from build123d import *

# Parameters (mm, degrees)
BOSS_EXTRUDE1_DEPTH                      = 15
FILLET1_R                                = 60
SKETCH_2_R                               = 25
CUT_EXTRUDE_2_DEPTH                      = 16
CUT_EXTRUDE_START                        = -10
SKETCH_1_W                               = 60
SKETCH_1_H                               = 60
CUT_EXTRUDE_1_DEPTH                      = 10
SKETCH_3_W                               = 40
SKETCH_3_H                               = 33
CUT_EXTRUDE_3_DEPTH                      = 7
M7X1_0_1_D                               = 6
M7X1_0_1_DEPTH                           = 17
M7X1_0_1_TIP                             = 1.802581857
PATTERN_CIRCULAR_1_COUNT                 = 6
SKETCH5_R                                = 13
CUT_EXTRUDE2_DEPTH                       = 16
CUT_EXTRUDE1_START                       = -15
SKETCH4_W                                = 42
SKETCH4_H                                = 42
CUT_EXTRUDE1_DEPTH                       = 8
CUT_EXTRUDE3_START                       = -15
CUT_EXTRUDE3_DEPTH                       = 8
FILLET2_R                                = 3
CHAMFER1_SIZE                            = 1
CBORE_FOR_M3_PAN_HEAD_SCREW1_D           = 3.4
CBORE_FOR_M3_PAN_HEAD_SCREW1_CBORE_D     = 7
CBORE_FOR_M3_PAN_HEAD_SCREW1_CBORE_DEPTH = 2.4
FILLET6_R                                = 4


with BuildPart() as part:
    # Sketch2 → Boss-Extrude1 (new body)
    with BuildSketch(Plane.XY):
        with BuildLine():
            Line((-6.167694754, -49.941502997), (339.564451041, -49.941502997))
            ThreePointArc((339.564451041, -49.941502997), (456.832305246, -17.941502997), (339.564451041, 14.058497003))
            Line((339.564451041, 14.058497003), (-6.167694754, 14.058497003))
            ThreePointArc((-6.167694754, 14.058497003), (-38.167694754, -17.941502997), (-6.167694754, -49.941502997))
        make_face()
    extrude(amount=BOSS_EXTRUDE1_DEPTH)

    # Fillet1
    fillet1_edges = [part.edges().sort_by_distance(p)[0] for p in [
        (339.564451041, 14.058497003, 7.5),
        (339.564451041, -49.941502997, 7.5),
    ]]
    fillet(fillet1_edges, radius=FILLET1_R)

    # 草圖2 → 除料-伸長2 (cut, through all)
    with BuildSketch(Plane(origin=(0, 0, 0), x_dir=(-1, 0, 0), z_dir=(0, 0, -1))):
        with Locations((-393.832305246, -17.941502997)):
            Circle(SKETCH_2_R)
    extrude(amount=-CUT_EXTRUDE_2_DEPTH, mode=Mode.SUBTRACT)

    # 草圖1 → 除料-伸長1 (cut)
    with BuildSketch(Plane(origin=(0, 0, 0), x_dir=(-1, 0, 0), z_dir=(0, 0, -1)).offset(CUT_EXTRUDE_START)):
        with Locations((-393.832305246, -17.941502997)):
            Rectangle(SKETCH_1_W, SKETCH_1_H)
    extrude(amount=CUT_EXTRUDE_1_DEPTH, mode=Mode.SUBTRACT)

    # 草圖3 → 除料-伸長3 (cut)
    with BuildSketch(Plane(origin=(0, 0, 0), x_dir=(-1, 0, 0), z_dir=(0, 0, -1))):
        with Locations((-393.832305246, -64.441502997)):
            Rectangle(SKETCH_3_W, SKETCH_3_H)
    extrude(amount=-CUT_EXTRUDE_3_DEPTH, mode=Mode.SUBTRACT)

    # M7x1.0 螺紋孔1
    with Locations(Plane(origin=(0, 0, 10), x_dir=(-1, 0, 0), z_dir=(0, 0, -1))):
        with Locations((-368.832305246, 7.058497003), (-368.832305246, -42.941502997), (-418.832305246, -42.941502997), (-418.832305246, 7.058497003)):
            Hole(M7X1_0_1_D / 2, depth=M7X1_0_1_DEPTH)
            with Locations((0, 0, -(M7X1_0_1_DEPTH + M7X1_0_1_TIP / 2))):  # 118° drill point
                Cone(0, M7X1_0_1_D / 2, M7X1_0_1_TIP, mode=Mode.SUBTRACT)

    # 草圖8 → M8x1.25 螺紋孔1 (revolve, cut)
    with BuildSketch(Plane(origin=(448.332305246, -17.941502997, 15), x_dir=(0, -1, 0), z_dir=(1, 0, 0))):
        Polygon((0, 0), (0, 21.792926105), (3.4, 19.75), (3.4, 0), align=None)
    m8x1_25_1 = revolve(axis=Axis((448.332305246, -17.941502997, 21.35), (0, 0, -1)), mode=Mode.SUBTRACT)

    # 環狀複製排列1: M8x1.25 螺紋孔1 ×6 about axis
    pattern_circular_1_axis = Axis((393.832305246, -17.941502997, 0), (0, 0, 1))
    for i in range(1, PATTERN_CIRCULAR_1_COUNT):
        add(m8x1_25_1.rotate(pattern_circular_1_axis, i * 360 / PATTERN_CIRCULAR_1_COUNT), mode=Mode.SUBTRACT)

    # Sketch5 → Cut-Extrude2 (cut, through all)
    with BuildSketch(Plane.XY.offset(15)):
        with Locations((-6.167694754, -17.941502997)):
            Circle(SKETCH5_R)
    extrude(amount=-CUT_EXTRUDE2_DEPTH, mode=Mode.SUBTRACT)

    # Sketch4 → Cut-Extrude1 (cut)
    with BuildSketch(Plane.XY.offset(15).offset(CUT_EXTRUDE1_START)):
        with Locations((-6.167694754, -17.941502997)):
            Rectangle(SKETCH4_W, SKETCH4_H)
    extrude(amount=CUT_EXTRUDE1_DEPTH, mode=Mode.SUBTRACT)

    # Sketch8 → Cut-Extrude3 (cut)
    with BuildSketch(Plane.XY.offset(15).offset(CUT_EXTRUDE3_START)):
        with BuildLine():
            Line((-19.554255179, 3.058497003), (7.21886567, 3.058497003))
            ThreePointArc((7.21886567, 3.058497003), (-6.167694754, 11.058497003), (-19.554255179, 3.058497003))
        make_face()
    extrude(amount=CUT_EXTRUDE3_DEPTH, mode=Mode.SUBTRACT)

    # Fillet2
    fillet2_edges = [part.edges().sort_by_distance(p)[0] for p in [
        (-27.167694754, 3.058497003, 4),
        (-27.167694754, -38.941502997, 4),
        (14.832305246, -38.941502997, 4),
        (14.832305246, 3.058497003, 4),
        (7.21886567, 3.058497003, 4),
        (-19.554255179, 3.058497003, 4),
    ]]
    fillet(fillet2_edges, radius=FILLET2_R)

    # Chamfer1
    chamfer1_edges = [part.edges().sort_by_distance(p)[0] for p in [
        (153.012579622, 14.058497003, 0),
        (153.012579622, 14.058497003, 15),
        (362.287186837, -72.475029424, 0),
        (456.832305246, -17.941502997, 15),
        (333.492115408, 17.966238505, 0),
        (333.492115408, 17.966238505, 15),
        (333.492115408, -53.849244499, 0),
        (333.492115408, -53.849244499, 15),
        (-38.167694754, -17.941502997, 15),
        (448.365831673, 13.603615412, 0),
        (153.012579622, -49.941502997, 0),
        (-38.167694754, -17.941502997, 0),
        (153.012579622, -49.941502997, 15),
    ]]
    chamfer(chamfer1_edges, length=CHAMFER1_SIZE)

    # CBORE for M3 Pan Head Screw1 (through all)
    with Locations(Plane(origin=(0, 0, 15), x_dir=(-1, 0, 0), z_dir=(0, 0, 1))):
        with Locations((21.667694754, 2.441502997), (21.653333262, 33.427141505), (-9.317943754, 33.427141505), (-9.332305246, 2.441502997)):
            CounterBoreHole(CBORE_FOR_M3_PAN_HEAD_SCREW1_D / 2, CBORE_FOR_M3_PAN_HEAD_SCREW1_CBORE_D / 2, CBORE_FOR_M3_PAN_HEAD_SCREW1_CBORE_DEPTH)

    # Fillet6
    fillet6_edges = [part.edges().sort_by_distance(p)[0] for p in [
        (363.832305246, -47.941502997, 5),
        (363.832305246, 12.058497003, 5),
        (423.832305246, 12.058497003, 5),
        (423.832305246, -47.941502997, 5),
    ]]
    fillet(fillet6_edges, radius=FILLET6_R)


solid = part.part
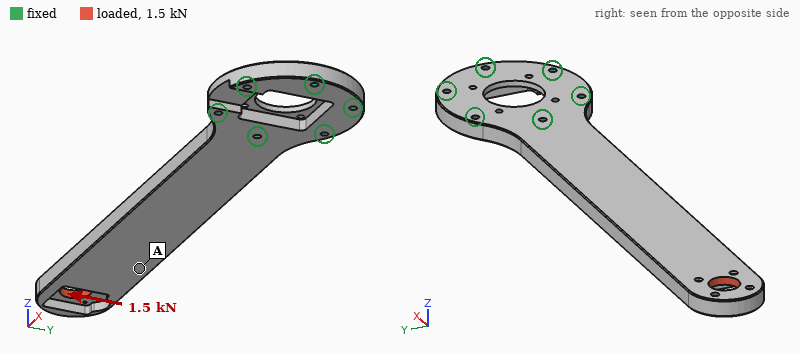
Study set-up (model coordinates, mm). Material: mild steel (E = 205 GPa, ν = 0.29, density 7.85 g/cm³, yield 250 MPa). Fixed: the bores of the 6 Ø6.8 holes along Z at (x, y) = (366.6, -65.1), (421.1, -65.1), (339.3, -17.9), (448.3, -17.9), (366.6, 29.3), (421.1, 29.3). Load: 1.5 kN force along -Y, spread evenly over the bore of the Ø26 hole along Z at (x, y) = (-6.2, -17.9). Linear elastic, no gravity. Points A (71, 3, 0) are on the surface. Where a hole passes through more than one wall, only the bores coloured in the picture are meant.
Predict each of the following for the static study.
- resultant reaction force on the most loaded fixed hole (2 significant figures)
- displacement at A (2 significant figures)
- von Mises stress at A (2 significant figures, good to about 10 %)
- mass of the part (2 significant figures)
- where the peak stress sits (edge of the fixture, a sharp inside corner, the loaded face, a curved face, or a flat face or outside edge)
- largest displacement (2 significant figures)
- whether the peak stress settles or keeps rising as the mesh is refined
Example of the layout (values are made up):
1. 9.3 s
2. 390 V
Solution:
1. 5.6 kN
2. 0.25 mm
3. 7.4 MPa
4. 3.6 kg
5. edge of the fixture
6. 0.41 mm
7. keeps rising
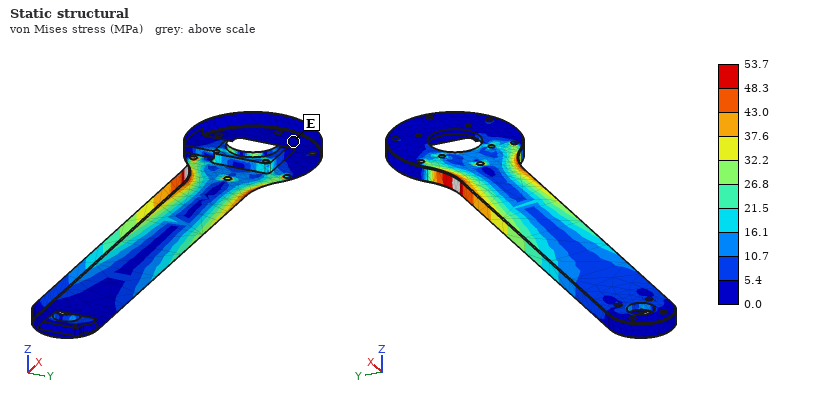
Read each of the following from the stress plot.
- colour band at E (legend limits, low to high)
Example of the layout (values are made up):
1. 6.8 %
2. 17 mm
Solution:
1. 0.0 to 5.4 MPa
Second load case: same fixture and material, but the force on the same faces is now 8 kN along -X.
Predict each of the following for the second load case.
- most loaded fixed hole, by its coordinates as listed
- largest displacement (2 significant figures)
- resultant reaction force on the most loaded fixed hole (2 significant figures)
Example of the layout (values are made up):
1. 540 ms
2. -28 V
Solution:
1. (339.3, -17.9)
2. 0.62 mm
3. 5.4 kN
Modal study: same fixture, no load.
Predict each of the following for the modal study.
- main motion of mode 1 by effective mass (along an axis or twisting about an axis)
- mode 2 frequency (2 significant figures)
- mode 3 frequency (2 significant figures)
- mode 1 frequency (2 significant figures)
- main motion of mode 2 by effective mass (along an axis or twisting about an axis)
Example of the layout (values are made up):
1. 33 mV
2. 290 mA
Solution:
1. along Z
2. 380 Hz
3. 580 Hz
4. 98 Hz
5. along Y
